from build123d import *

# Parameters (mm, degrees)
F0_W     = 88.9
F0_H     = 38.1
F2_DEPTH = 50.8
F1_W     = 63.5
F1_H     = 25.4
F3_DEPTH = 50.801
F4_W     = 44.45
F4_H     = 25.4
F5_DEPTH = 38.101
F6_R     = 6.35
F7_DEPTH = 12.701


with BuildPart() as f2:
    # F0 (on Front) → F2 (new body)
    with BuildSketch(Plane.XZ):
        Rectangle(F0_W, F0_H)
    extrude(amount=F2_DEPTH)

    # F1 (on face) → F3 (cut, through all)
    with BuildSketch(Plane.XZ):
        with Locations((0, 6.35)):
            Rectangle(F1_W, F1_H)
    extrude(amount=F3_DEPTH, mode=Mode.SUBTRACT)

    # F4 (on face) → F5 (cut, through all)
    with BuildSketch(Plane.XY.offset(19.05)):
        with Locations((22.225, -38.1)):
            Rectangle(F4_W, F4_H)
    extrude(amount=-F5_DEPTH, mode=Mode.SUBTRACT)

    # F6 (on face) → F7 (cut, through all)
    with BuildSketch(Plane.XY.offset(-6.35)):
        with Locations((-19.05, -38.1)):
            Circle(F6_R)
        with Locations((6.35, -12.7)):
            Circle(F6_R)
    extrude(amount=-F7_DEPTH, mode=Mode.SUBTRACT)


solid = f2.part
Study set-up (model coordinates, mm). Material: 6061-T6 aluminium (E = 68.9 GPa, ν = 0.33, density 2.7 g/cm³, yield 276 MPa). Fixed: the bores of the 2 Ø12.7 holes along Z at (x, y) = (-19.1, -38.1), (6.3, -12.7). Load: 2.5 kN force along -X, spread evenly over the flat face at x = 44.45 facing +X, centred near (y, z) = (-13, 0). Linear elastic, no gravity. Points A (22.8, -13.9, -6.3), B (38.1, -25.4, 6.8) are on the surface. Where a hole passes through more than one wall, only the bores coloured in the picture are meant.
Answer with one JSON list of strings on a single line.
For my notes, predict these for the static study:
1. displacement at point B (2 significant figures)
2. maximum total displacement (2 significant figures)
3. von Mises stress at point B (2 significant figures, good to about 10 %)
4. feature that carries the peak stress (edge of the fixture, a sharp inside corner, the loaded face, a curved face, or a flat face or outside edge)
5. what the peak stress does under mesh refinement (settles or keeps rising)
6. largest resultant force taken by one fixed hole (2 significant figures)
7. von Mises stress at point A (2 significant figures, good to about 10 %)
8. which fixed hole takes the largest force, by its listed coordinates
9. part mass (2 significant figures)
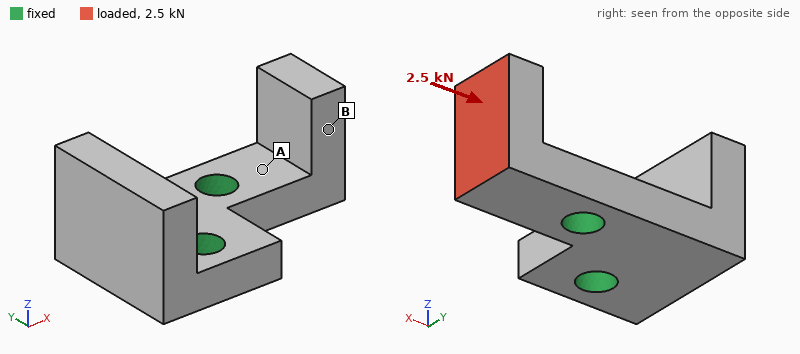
["0.077 mm", "0.13 mm", "8.7 MPa", "edge of the fixture", "keeps rising", "2.5 kN", "56 MPa", "(6.3, -12.7)", "170 g"]
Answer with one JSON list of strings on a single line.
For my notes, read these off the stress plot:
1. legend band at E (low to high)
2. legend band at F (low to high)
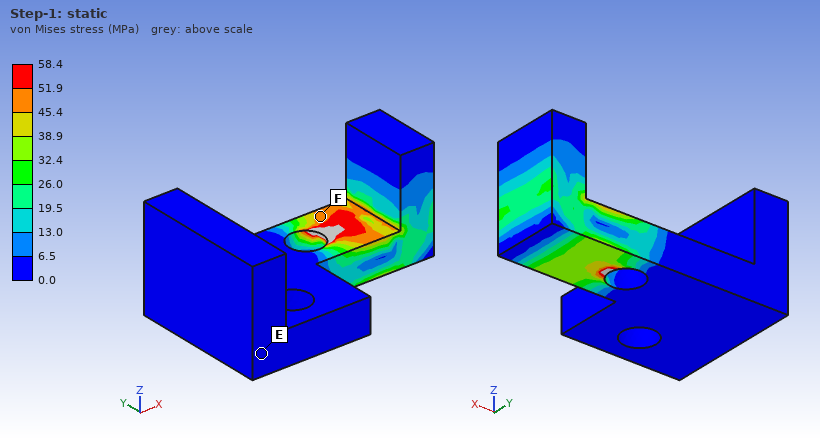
["0.0 to 6.5 MPa", "45.4 to 51.9 MPa"]
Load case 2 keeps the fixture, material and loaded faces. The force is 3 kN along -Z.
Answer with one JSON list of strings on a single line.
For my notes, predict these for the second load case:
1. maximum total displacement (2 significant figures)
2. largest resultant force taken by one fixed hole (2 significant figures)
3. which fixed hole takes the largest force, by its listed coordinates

["0.24 mm", "3.1 kN", "(6.3, -12.7)"]
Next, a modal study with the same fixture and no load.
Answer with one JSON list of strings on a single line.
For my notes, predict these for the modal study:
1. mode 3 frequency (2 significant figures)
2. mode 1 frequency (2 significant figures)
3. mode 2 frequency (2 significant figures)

["4700 Hz", "3800 Hz", "4700 Hz"]
